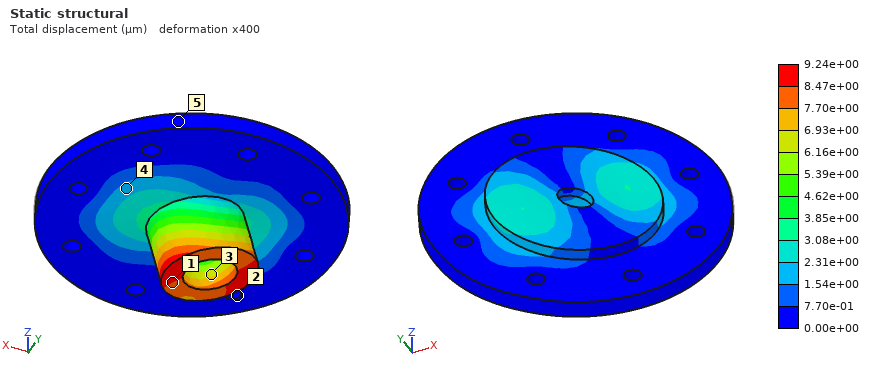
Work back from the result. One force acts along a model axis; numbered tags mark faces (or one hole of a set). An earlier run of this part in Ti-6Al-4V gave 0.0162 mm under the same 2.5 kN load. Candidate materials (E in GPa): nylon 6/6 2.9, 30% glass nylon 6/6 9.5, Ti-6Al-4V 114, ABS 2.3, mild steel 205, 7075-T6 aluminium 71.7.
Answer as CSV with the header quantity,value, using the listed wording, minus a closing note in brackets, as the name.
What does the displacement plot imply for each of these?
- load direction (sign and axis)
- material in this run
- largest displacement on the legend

quantity,value
load direction,-X
material in this run,mild steel
largest displacement on the legend,9.24e+00 µm
